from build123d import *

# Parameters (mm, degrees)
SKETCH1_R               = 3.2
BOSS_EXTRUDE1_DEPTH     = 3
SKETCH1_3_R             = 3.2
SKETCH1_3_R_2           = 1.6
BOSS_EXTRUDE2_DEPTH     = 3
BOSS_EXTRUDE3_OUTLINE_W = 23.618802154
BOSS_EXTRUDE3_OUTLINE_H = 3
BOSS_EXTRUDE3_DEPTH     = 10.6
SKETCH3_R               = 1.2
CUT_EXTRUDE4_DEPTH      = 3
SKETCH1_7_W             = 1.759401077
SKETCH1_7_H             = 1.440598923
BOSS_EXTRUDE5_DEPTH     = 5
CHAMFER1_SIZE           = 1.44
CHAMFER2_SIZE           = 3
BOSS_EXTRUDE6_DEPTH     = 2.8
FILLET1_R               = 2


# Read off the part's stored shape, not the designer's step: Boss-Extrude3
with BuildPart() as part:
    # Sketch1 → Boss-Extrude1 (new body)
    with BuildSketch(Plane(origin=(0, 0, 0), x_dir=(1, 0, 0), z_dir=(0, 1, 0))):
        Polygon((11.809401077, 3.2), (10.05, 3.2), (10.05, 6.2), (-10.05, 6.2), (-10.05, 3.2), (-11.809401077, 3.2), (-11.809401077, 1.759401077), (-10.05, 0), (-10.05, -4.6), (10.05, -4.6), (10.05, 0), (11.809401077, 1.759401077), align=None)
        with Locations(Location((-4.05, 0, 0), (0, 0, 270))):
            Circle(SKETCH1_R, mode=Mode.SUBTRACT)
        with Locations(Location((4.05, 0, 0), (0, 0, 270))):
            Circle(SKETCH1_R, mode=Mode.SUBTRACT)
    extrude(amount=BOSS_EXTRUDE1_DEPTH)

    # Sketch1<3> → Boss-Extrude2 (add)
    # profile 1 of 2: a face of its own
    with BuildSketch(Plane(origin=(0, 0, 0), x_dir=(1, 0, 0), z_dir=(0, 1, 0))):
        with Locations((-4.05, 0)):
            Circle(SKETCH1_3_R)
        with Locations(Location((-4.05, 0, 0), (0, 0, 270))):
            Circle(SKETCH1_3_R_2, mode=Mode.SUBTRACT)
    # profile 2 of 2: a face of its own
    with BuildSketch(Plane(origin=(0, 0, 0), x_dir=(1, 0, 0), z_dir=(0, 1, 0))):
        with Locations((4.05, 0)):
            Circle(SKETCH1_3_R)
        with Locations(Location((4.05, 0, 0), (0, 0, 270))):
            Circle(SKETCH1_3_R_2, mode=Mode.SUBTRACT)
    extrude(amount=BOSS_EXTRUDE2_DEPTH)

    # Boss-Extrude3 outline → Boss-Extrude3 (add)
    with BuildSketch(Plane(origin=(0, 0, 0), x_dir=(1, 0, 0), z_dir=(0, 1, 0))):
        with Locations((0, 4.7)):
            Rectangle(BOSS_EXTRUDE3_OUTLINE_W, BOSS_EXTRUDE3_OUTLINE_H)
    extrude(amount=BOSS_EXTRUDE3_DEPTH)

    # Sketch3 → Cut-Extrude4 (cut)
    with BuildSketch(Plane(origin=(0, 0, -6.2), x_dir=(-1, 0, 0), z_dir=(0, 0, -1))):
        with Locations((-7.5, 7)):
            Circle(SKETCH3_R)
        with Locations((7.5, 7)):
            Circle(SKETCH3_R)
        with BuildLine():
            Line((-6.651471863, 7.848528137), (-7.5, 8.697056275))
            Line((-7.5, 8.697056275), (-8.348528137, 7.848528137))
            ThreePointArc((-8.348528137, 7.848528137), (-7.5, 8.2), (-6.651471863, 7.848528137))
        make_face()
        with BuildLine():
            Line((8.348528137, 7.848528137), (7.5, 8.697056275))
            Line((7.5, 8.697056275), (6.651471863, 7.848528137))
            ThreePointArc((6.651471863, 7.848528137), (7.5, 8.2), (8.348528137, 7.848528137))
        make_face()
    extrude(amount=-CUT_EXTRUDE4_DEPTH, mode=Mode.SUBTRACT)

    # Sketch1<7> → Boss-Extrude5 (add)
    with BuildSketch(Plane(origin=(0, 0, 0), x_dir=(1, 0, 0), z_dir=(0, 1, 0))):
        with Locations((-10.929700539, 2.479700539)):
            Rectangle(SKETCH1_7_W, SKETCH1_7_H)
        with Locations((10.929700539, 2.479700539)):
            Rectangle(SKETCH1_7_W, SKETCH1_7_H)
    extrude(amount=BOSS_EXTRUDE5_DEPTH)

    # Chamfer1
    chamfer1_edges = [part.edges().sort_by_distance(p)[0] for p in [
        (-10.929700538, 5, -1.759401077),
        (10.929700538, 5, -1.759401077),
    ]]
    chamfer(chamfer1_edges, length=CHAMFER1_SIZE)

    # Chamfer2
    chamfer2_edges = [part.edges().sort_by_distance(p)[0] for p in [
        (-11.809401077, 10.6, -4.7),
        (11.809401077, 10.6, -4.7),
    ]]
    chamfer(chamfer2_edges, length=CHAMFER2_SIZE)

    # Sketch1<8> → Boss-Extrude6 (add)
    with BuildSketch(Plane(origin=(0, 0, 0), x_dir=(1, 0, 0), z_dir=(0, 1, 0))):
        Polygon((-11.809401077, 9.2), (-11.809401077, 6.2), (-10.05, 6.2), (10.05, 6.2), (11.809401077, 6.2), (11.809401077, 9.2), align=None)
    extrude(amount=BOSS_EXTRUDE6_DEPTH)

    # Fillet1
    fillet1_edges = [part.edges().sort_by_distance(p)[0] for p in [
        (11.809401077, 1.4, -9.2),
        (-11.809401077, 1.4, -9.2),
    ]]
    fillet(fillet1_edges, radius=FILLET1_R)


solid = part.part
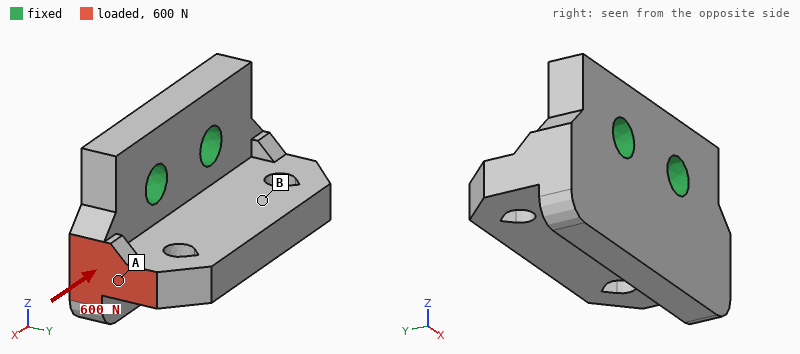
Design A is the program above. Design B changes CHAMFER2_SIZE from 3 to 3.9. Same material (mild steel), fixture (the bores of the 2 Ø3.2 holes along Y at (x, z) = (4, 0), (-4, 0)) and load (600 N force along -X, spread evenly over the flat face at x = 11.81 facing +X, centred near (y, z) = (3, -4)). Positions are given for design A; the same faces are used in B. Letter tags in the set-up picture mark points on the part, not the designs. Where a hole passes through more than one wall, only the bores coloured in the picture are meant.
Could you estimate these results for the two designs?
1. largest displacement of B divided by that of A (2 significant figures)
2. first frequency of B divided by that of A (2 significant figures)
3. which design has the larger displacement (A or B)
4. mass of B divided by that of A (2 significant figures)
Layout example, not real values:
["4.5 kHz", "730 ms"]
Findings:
["0.90", "1.0", "A", "0.99"]
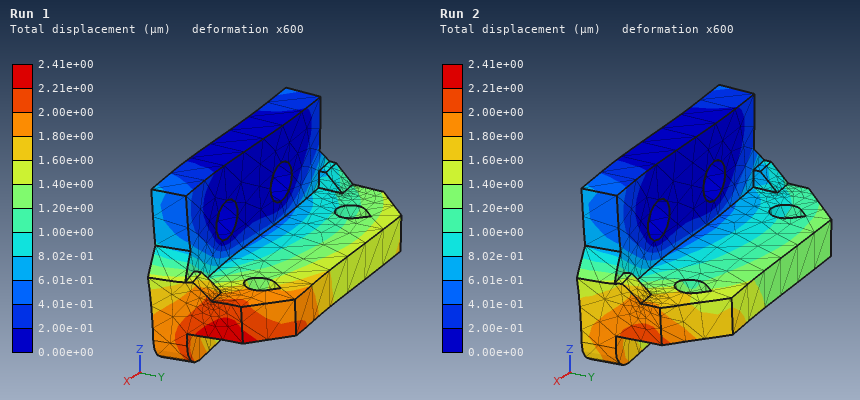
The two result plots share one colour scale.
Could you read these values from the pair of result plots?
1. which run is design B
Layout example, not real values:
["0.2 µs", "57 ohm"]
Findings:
["Run 2"]
